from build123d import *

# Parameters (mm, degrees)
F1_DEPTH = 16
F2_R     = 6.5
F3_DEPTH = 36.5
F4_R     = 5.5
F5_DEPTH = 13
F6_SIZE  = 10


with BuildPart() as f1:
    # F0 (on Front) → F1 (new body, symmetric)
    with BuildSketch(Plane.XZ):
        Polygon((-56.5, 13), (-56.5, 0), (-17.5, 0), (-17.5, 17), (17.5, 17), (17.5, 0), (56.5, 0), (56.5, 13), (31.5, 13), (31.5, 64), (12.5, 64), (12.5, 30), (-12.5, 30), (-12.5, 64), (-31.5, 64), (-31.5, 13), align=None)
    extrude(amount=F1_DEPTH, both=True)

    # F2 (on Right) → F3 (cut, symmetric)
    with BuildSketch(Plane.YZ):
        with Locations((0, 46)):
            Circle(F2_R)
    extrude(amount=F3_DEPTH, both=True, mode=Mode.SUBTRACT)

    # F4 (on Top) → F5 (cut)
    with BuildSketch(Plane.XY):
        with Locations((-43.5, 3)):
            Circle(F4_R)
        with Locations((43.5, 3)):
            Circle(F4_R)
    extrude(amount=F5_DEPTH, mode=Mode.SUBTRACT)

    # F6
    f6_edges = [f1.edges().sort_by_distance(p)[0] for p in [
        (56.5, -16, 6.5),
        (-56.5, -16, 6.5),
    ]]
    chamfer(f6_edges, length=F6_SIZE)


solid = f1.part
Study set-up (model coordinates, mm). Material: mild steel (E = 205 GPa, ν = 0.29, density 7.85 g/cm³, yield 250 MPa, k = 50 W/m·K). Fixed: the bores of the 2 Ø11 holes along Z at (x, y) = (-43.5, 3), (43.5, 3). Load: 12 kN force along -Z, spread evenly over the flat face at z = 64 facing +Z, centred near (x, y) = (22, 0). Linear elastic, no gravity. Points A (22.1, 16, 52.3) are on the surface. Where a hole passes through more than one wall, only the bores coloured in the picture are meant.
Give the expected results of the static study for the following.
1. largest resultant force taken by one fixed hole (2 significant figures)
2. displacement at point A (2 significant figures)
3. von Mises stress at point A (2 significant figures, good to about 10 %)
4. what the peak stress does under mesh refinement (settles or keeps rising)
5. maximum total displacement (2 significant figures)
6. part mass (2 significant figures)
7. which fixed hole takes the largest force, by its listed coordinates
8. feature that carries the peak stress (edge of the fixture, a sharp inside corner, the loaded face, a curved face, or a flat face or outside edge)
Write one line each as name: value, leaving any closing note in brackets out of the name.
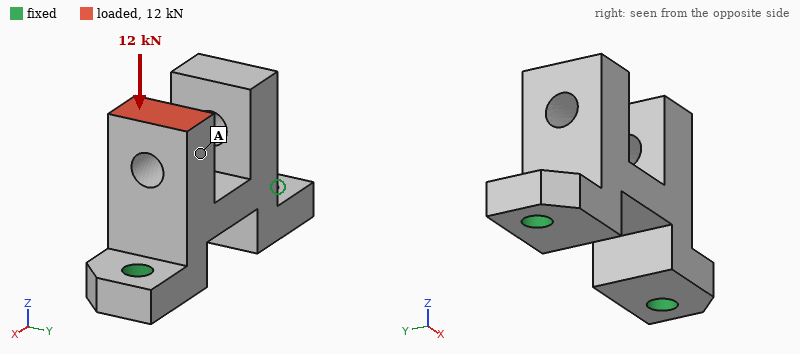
largest resultant force taken by one fixed hole: 11 kN
displacement at point A: 14 µm
von Mises stress at point A: 19 MPa
what the peak stress does under mesh refinement: keeps rising
maximum total displacement: 20 µm
part mass: 740 g
which fixed hole takes the largest force, by its listed coordinates: (43.5, 3)
feature that carries the peak stress: edge of the fixture
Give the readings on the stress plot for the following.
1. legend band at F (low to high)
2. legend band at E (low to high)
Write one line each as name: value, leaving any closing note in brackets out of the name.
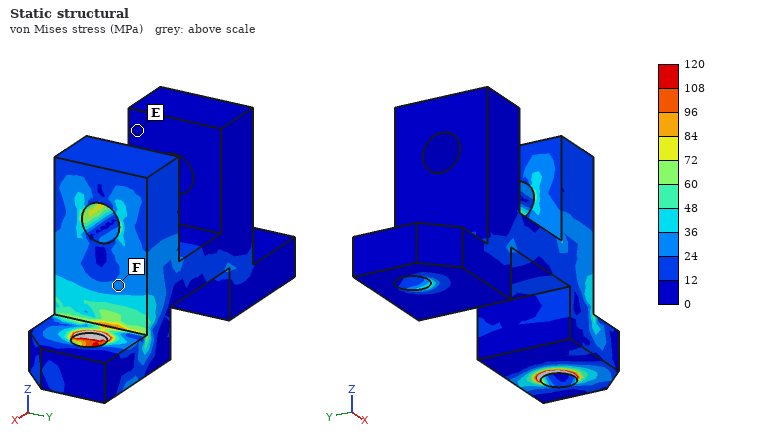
legend band at F: 24 to 36 MPa
legend band at E: 0 to 12 MPa
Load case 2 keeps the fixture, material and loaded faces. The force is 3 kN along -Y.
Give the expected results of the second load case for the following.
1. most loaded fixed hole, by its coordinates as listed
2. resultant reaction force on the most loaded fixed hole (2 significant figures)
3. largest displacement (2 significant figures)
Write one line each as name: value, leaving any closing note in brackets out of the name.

most loaded fixed hole, by its coordinates as listed: (43.5, 3)
resultant reaction force on the most loaded fixed hole: 2.1 kN
largest displacement: 84 µm
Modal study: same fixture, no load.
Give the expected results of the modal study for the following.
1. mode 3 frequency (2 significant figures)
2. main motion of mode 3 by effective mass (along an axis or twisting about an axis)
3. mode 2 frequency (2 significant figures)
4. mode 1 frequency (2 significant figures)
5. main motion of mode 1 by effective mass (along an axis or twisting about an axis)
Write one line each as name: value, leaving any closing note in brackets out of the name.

mode 3 frequency: 5500 Hz
main motion of mode 3 by effective mass: along X
mode 2 frequency: 4500 Hz
mode 1 frequency: 2800 Hz
main motion of mode 1 by effective mass: along Y
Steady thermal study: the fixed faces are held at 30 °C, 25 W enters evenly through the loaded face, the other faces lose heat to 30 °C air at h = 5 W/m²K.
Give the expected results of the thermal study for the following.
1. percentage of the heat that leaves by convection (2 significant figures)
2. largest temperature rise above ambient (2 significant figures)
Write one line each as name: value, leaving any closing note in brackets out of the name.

percentage of the heat that leaves by convection: 6.4 %
largest temperature rise above ambient: 61 K
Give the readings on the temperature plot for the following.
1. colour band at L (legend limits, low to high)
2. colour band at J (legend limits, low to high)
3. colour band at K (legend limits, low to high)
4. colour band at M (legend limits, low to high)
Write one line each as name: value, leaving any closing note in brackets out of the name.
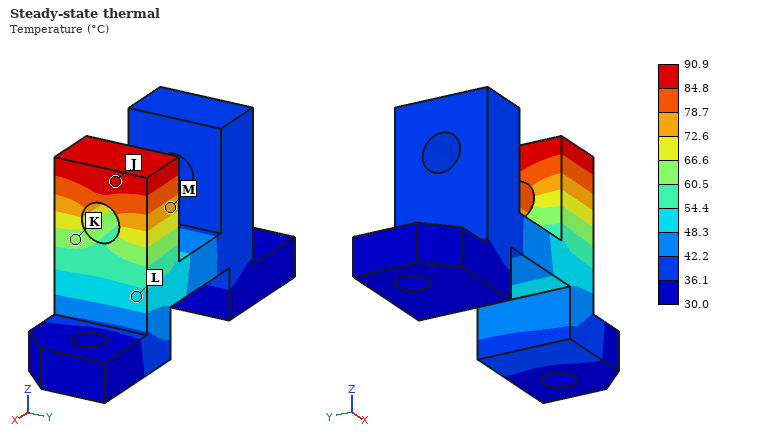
colour band at L: 48.3 to 54.4 °C
colour band at J: 84.8 to 90.9 °C
colour band at K: 60.5 to 66.6 °C
colour band at M: 72.6 to 78.7 °C
